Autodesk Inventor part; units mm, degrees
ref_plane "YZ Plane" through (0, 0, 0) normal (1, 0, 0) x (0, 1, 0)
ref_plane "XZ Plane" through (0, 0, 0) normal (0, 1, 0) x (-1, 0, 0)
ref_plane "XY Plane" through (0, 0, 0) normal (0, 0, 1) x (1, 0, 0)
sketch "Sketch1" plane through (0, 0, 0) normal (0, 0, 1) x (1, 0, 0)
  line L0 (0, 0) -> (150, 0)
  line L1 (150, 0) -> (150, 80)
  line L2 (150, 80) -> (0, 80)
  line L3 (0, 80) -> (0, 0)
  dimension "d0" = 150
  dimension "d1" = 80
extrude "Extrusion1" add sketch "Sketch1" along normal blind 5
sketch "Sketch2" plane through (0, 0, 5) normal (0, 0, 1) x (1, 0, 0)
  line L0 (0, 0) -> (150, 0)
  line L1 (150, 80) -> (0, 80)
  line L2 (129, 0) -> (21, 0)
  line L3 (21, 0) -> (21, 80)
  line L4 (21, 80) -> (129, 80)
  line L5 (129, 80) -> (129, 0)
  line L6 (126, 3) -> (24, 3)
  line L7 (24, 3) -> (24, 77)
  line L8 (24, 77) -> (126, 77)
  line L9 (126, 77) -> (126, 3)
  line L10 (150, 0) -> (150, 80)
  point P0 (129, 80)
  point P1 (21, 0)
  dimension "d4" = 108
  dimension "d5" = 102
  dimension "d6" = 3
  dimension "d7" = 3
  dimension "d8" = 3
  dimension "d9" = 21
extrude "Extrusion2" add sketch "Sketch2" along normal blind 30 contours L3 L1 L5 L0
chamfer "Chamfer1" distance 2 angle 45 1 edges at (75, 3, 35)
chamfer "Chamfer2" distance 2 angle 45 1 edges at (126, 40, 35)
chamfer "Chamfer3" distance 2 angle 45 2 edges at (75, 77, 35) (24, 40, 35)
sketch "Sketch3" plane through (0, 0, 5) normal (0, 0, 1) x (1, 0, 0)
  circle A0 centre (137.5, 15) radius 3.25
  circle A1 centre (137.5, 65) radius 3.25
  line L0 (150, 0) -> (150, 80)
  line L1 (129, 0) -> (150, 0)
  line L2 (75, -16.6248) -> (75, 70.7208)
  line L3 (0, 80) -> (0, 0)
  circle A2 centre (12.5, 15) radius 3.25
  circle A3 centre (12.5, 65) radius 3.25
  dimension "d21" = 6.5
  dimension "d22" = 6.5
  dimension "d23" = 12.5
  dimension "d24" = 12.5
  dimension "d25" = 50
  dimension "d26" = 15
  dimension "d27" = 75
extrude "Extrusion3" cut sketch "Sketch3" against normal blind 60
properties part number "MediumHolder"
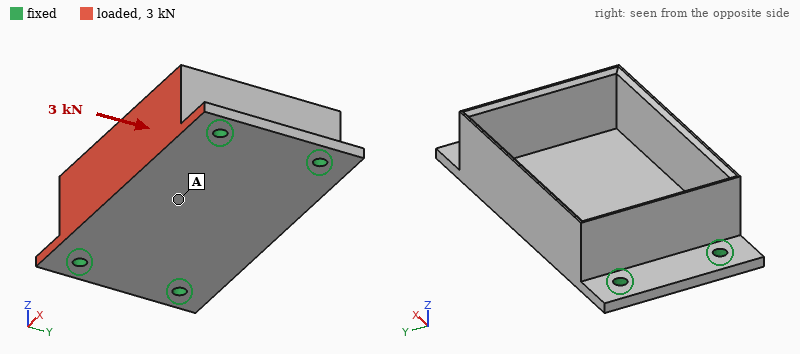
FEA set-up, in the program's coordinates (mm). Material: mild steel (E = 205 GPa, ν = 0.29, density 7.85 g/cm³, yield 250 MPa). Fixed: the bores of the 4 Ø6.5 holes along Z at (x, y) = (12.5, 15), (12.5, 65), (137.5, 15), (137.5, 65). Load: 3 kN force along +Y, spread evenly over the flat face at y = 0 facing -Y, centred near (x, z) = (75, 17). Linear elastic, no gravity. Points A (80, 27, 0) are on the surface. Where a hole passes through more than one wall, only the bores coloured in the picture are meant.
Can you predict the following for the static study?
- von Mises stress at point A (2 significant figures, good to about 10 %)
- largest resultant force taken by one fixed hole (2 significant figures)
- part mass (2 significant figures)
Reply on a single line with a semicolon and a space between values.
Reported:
17 MPa; 1.1 kN; 720 g
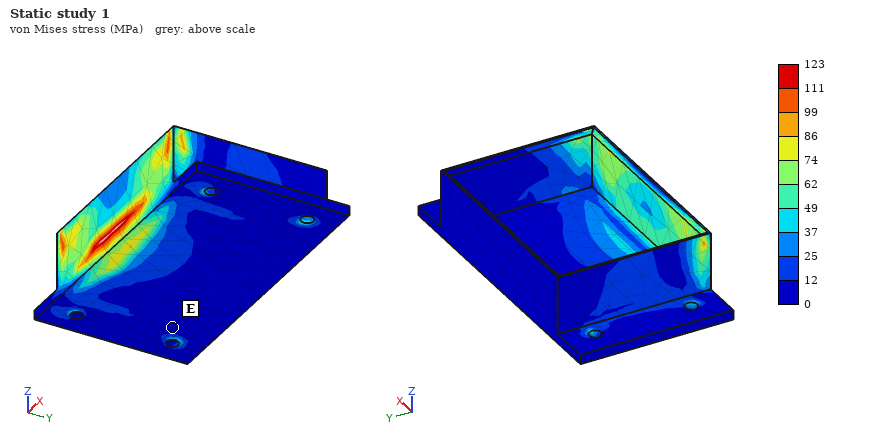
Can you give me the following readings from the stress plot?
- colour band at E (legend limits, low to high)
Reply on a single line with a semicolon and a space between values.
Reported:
0 to 12 MPa
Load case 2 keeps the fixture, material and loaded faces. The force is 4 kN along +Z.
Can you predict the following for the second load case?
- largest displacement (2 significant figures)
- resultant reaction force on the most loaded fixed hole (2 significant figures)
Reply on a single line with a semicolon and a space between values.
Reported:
64 µm; 2.9 kN
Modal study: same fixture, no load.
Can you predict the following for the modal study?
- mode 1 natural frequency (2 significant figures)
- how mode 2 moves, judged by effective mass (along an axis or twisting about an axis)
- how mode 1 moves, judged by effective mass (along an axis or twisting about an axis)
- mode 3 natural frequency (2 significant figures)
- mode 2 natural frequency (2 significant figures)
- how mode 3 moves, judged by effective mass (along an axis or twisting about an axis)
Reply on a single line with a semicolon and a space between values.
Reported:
2700 Hz; along Y; along Z; 3300 Hz; 3000 Hz; along Z
